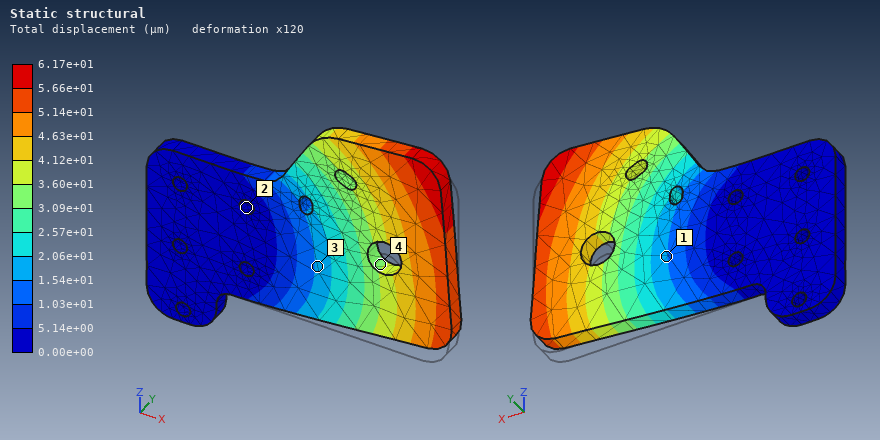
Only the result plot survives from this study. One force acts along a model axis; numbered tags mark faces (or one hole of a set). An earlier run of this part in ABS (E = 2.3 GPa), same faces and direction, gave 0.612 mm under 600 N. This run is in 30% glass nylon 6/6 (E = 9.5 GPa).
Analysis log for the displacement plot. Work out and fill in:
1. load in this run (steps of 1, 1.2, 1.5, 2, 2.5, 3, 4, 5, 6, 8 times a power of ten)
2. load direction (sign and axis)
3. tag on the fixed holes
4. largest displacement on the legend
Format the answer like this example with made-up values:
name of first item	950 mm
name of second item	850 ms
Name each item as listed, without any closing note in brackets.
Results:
load in this run	250 N
load direction	+Z
tag on the fixed holes	2
largest displacement on the legend	6.17e+01 µm
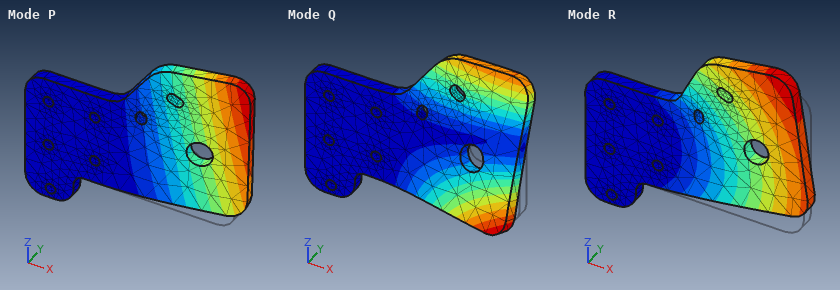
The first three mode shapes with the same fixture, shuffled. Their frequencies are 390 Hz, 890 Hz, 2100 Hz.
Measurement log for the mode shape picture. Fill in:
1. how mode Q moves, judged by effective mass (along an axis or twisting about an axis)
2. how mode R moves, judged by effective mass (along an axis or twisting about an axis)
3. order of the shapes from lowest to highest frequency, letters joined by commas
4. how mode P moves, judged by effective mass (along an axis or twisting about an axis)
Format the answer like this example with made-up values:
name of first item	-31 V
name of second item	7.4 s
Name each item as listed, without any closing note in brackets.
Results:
how mode Q moves, judged by effective mass	twisting about X
how mode R moves, judged by effective mass	along Z
order of the shapes from lowest to highest frequency, letters joined by commas	P, Q, R
how mode P moves, judged by effective mass	along Y
